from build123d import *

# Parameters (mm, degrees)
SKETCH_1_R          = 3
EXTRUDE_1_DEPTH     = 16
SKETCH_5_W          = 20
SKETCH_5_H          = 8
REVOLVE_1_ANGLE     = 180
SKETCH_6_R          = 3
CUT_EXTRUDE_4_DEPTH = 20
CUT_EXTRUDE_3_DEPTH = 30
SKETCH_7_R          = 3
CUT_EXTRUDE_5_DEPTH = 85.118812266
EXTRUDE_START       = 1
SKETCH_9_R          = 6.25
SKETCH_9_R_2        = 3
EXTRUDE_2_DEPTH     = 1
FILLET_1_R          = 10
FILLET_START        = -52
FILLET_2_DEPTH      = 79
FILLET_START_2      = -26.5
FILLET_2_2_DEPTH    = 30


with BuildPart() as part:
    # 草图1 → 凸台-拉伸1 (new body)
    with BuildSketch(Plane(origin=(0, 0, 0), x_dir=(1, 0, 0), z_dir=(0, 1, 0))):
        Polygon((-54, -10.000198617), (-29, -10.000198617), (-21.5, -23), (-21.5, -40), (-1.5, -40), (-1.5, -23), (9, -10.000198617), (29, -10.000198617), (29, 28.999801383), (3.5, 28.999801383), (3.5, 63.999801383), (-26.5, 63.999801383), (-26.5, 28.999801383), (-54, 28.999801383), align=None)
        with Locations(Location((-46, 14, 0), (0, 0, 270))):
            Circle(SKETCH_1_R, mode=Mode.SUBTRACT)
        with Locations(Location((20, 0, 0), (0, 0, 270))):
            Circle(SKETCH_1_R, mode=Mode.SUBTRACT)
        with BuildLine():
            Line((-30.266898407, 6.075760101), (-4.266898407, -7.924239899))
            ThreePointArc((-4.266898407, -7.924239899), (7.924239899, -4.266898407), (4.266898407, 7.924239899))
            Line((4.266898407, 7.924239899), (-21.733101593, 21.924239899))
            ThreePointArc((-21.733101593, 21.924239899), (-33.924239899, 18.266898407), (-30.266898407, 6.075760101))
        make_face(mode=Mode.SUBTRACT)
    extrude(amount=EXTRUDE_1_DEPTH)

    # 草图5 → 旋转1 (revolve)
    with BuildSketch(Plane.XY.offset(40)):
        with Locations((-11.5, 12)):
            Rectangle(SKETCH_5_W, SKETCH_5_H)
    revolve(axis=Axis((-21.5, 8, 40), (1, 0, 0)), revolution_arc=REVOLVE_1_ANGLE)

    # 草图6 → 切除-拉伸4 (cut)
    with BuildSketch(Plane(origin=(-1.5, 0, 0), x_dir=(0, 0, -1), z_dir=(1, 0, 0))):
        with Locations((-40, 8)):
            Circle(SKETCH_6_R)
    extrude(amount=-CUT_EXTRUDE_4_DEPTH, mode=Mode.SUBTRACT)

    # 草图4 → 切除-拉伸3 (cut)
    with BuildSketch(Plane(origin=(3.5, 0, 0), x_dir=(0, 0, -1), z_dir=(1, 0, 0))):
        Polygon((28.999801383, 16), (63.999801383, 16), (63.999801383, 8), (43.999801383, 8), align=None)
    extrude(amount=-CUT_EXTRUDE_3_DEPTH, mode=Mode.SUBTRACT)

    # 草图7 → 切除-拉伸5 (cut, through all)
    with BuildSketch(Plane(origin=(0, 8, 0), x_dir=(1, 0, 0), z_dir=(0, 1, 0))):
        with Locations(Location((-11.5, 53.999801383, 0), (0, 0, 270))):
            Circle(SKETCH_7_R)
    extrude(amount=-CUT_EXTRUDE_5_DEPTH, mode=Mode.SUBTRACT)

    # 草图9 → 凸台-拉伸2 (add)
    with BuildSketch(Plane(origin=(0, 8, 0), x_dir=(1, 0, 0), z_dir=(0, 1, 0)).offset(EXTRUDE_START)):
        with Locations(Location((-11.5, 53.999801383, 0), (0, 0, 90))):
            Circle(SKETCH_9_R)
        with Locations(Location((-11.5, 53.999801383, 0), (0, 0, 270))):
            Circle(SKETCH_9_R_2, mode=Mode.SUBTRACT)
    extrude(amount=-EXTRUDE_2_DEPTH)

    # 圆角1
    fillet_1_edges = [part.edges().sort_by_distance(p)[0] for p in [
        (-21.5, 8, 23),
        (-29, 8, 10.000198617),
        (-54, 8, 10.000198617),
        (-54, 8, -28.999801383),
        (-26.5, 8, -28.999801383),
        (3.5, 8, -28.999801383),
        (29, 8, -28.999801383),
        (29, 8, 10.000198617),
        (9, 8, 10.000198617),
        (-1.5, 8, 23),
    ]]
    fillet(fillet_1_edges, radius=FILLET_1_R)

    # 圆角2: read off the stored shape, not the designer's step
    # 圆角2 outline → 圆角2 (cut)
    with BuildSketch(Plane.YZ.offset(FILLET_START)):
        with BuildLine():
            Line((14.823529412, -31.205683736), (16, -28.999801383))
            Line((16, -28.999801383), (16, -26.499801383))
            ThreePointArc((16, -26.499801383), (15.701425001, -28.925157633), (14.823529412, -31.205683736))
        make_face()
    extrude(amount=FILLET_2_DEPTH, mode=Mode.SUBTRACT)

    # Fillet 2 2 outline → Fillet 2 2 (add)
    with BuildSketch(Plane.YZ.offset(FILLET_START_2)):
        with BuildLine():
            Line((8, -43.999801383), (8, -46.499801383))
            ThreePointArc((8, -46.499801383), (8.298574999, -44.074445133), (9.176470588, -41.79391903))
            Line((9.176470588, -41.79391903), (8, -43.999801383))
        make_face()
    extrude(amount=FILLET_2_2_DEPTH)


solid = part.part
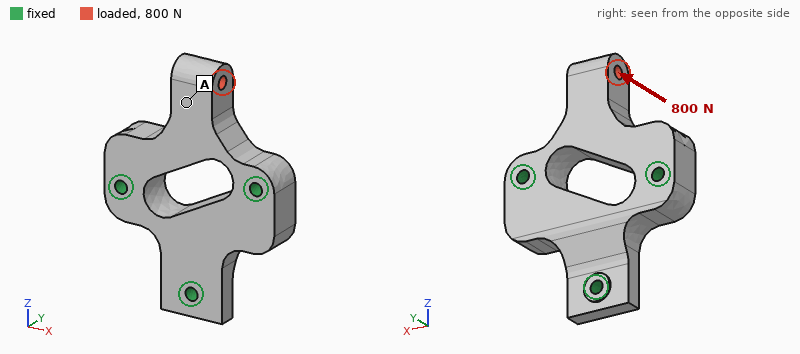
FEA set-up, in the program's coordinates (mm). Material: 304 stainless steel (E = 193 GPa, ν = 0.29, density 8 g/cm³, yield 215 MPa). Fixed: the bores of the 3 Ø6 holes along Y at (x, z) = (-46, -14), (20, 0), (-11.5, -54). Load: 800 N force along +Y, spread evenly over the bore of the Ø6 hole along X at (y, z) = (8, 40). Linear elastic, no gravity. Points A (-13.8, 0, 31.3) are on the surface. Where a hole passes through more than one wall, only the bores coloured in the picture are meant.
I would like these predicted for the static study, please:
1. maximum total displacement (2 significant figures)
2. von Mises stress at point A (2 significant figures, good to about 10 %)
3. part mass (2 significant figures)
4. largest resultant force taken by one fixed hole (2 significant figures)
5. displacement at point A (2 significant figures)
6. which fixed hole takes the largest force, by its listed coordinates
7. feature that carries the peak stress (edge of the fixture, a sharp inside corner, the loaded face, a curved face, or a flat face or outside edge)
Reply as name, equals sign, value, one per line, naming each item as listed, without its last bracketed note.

maximum total displacement = 40 µm
von Mises stress at point A = 8.6 MPa
part mass = 490 g
largest resultant force taken by one fixed hole = 610 N
displacement at point A = 25 µm
which fixed hole takes the largest force, by its listed coordinates = (20, 0)
feature that carries the peak stress = a curved face
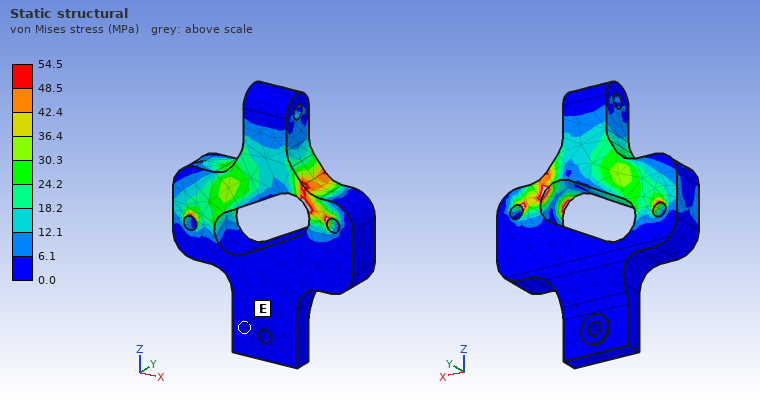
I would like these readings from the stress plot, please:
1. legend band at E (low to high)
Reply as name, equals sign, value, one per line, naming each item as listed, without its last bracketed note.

legend band at E = 0.0 to 6.1 MPa
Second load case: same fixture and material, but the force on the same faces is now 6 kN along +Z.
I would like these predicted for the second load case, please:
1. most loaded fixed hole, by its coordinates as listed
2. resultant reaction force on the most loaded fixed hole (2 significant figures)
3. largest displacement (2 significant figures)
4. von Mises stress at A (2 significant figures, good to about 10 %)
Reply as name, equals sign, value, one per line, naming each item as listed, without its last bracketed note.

most loaded fixed hole, by its coordinates as listed = (-46, -14)
resultant reaction force on the most loaded fixed hole = 4.1 kN
largest displacement = 10 µm
von Mises stress at A = 19 MPa
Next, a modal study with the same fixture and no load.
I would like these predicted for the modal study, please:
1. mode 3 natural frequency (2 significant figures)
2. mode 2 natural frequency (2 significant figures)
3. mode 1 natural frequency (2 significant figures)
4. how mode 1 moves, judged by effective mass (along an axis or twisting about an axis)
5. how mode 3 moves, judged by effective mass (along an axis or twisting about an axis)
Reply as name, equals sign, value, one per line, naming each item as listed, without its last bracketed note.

mode 3 natural frequency = 12 kHz
mode 2 natural frequency = 10 kHz
mode 1 natural frequency = 3600 Hz
how mode 1 moves, judged by effective mass = along Y
how mode 3 moves, judged by effective mass = along Y
